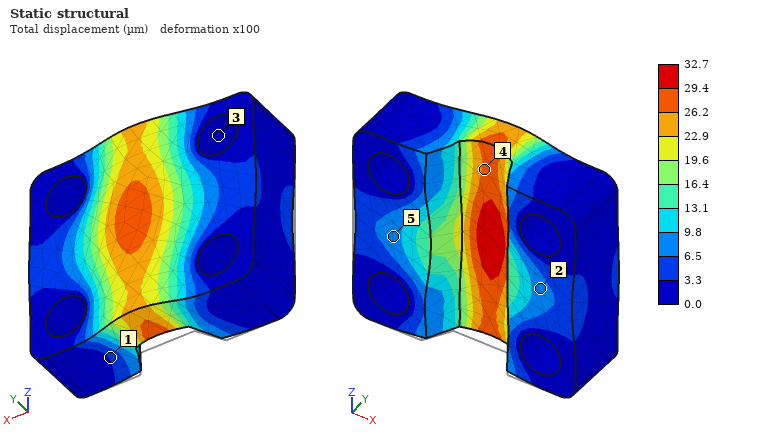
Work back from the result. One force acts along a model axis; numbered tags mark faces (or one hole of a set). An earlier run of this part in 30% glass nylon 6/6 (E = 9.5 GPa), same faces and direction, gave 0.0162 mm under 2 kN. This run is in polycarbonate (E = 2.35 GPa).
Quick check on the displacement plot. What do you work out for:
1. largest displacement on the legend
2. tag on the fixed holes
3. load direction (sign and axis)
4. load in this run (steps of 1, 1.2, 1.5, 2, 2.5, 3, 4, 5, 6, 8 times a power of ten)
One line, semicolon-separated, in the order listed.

32.7 µm; 3; +Y; 1 kN
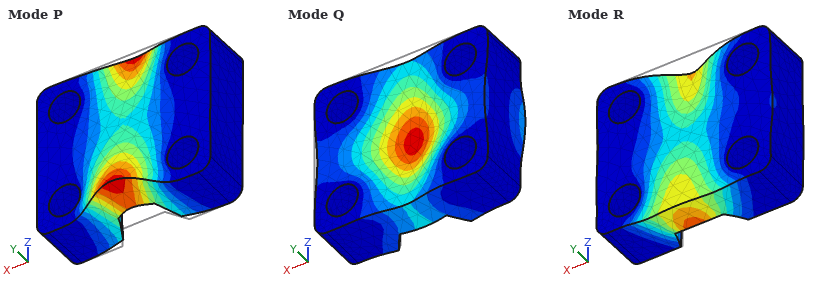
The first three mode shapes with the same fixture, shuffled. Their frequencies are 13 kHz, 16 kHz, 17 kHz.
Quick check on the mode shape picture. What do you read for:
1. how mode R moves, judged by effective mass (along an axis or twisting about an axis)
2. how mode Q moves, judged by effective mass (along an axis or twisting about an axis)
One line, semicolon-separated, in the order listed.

along Z; along Y
